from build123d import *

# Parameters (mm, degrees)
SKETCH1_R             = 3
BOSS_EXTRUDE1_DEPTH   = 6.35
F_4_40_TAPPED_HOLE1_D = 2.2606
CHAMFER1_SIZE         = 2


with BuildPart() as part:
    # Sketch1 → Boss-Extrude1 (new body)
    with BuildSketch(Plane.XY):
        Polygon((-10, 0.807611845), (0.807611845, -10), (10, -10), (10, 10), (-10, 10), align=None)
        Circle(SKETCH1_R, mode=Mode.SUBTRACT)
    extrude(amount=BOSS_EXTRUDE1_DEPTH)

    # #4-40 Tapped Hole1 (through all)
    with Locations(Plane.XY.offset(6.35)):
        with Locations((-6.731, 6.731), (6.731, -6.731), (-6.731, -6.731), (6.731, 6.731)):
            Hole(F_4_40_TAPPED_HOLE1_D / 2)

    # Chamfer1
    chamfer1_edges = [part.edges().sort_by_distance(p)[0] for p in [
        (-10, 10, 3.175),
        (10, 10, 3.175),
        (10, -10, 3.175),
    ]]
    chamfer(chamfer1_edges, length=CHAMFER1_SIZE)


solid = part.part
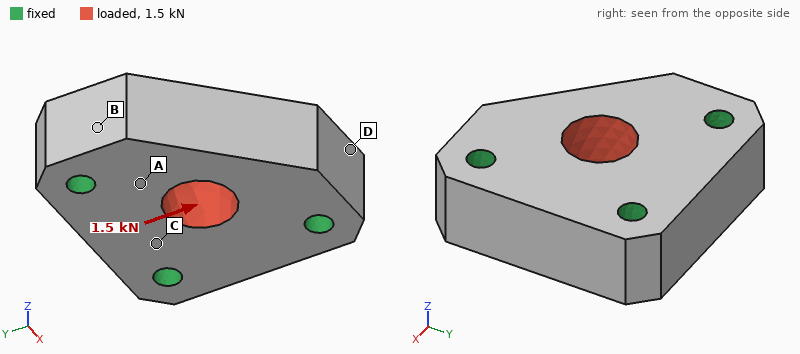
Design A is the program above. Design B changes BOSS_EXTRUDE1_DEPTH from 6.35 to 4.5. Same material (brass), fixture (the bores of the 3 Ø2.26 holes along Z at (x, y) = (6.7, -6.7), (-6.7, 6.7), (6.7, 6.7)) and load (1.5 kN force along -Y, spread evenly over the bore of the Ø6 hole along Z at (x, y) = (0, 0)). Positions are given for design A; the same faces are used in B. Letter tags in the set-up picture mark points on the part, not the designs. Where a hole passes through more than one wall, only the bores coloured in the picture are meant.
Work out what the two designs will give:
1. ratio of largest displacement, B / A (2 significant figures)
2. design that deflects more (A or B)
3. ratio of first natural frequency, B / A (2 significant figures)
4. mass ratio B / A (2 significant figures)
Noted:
1.4
B
0.83
0.71
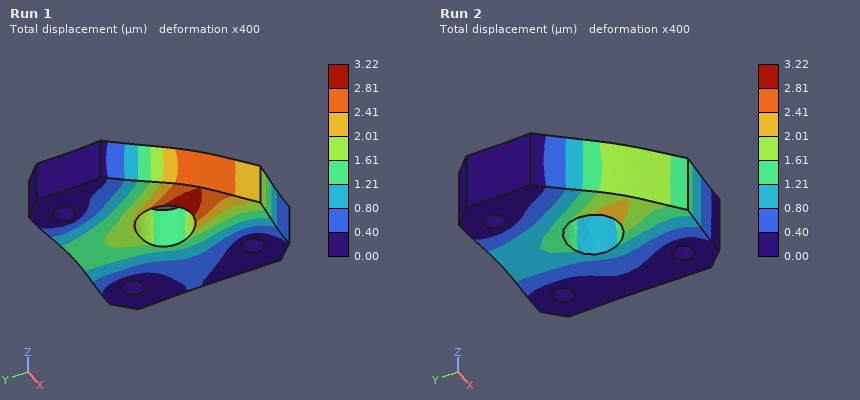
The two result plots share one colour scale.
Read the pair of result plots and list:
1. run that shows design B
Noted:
Run 1
